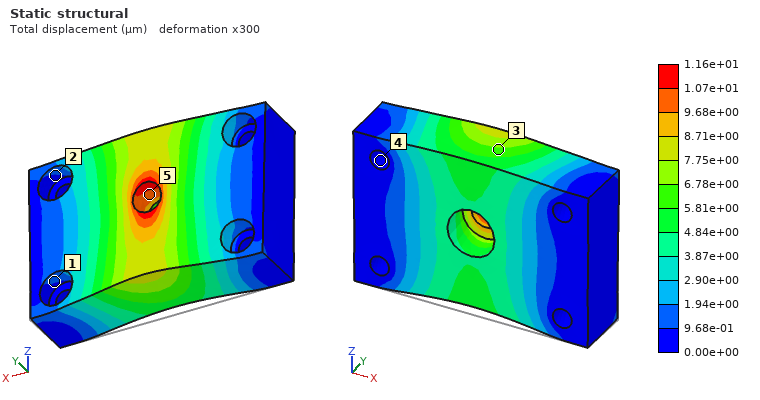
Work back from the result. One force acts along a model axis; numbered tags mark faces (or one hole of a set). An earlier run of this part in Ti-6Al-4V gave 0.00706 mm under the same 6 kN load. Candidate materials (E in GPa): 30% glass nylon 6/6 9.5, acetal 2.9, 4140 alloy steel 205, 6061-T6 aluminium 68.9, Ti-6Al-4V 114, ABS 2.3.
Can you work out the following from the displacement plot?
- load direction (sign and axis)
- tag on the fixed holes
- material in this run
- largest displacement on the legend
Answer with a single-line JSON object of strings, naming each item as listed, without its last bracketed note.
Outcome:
{"load direction": "+Z", "tag on the fixed holes": "4", "material in this run": "6061-T6 aluminium", "largest displacement on the legend": "1.16e+01 µm"}
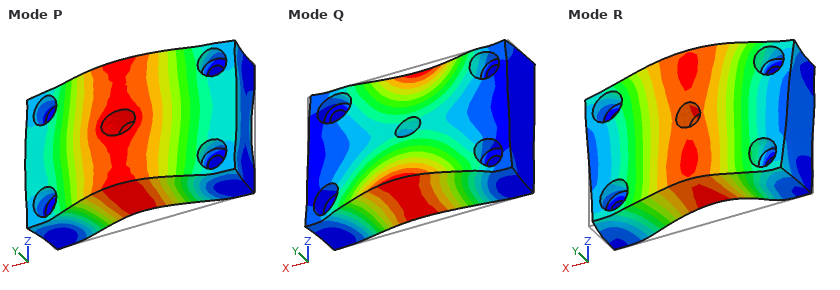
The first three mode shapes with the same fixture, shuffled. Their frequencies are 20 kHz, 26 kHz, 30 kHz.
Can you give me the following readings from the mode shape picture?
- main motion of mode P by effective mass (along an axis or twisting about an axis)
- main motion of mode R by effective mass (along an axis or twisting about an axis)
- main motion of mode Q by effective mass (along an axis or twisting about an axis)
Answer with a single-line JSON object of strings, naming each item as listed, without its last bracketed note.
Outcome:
{"main motion of mode P by effective mass": "along Y", "main motion of mode R by effective mass": "along Z", "main motion of mode Q by effective mass": "twisting about X"}
